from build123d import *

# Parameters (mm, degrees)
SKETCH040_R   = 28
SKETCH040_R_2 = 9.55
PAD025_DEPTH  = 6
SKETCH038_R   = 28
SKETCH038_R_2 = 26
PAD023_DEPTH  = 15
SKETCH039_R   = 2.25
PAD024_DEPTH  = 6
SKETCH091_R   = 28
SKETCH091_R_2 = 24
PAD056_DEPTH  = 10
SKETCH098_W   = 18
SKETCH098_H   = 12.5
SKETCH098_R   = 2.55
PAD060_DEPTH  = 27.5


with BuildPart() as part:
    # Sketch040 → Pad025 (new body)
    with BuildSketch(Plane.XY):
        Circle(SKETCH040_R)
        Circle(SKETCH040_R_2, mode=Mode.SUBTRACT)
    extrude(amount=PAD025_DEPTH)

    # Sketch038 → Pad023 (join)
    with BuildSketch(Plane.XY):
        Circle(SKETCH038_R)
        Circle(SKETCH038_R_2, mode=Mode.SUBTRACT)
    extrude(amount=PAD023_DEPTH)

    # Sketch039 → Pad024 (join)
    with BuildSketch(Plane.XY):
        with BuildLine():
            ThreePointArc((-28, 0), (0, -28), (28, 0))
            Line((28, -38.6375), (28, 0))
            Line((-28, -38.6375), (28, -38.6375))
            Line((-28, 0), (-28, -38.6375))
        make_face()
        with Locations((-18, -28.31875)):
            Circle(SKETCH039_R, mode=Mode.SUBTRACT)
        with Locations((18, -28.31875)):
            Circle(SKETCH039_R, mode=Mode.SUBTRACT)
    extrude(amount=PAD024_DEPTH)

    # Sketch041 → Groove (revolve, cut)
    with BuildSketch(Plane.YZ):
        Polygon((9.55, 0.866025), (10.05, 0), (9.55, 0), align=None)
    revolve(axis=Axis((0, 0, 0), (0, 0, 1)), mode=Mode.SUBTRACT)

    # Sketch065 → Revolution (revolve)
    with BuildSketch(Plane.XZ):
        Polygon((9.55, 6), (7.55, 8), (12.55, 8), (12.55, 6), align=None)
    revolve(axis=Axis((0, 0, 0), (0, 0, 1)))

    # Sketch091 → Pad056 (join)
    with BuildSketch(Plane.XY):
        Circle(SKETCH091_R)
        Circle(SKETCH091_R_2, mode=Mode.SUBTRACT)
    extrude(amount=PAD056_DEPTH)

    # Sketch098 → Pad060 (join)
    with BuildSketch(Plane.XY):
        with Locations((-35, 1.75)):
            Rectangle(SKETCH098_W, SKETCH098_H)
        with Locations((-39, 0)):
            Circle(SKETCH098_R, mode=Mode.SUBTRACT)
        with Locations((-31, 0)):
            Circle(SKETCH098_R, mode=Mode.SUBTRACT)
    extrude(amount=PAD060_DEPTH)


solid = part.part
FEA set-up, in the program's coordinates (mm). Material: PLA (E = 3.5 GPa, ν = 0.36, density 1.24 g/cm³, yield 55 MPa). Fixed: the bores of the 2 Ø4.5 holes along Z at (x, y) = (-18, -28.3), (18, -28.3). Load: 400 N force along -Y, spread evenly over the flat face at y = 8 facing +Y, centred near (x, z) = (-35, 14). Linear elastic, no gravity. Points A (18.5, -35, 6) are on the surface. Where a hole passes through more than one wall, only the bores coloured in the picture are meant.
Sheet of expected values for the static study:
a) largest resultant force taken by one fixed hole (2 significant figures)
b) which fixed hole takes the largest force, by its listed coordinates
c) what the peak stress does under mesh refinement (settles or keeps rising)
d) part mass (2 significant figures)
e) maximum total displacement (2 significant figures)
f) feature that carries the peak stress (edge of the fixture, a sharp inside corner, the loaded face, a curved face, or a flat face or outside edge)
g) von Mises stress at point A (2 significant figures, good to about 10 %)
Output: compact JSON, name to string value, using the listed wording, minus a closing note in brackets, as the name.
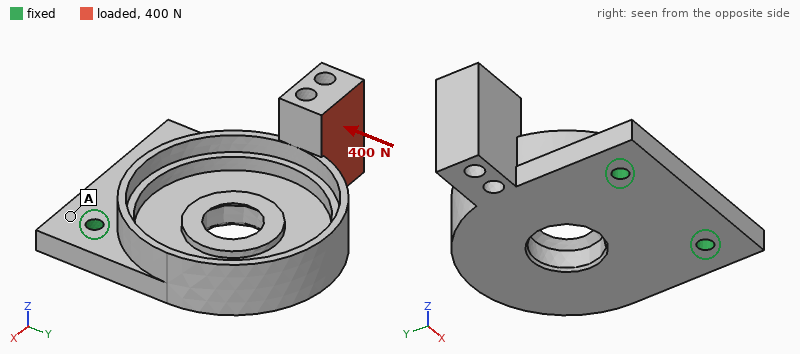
{"largest resultant force taken by one fixed hole": "570 N", "which fixed hole takes the largest force, by its listed coordinates": "(-18, -28.3)", "what the peak stress does under mesh refinement": "keeps rising", "part mass": "35 g", "maximum total displacement": "1.2 mm", "feature that carries the peak stress": "edge of the fixture", "von Mises stress at point A": "3.7 MPa"}
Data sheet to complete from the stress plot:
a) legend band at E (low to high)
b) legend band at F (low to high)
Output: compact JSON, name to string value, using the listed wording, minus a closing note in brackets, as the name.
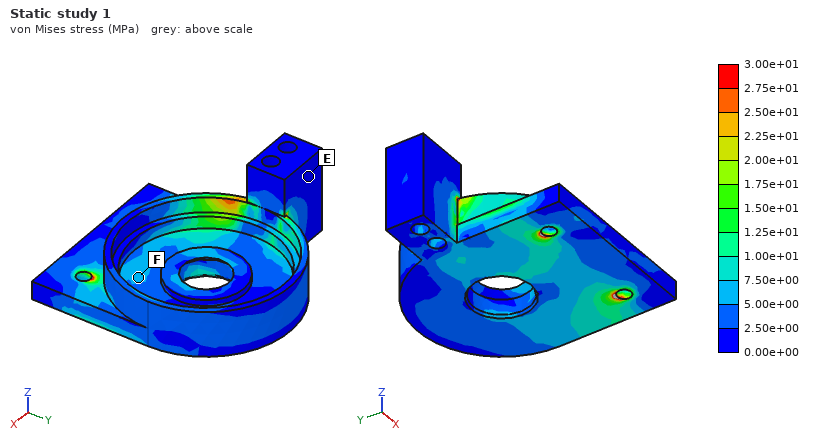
{"legend band at E": "0.00e+00 to 2.50e+00 MPa", "legend band at F": "5.00e+00 to 7.50e+00 MPa"}
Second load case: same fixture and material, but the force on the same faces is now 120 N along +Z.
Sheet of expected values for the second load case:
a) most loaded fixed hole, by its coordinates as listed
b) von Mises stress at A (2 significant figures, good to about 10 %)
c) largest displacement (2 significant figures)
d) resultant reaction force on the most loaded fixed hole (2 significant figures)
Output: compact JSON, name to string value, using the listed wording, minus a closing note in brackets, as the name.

{"most loaded fixed hole, by its coordinates as listed": "(-18, -28.3)", "von Mises stress at A": "2.8 MPa", "largest displacement": "1.2 mm", "resultant reaction force on the most loaded fixed hole": "170 N"}
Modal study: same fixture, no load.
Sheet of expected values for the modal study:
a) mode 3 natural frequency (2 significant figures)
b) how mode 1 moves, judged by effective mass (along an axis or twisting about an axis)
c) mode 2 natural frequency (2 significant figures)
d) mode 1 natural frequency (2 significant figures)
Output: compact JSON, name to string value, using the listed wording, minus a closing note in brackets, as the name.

{"mode 3 natural frequency": "1800 Hz", "how mode 1 moves, judged by effective mass": "along Z", "mode 2 natural frequency": "870 Hz", "mode 1 natural frequency": "500 Hz"}
